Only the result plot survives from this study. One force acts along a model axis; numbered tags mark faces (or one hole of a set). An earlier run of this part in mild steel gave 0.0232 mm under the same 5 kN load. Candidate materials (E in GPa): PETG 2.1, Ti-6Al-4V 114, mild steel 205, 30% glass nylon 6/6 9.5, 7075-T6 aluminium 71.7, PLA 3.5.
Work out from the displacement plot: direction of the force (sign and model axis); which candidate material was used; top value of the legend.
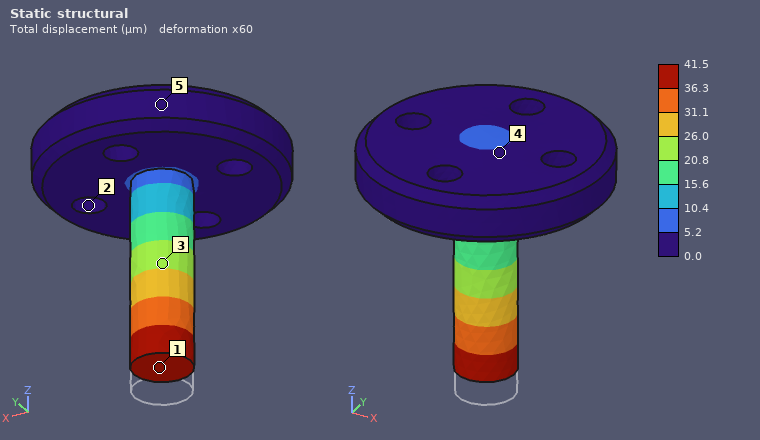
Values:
+Z
Ti-6Al-4V
41.5 µm
